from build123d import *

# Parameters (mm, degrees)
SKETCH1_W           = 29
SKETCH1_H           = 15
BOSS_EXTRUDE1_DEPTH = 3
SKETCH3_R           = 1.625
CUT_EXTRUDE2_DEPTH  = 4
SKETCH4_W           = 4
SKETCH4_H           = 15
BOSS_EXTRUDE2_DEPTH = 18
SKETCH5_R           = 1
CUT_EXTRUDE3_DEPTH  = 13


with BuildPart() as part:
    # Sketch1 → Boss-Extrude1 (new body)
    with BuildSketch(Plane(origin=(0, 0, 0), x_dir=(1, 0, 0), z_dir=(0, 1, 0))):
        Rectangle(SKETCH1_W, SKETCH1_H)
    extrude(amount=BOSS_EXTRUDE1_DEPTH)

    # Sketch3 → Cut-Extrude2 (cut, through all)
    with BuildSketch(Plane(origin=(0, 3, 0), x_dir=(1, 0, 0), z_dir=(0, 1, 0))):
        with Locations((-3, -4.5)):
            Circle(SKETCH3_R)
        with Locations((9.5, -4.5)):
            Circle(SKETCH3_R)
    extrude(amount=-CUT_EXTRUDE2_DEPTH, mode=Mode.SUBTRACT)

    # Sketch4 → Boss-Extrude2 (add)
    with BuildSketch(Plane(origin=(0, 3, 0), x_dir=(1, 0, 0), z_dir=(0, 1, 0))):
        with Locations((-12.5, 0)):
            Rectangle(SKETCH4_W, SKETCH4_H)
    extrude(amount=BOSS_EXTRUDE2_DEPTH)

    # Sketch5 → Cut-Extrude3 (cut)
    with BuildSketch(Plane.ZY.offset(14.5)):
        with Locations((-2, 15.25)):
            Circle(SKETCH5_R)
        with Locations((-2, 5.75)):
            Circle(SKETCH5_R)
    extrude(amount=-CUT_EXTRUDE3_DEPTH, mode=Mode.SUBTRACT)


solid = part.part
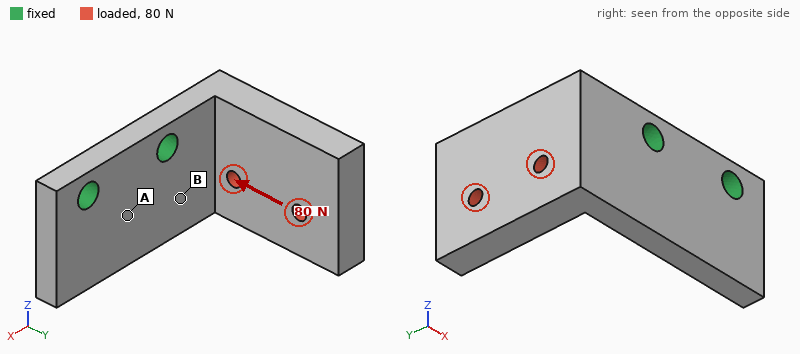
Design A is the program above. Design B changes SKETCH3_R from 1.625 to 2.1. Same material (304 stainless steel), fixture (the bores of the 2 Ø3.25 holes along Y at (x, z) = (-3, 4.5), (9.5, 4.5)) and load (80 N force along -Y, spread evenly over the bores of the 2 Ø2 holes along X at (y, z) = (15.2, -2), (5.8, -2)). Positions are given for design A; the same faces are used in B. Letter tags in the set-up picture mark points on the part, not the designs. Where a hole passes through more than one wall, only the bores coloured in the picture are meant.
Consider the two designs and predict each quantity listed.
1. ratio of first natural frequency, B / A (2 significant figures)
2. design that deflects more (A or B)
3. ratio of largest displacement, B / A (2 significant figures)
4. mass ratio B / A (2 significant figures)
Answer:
1.0
A
0.88
0.99
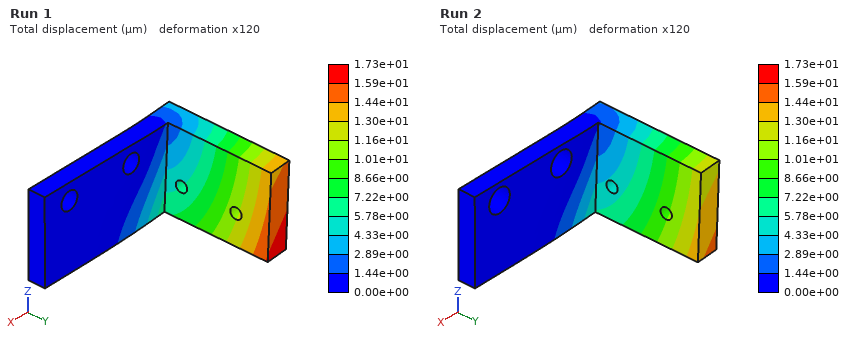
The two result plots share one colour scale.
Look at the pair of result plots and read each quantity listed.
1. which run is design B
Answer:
Run 2
